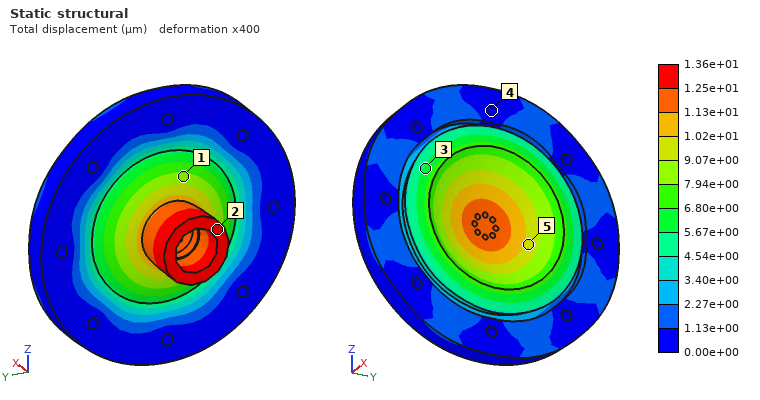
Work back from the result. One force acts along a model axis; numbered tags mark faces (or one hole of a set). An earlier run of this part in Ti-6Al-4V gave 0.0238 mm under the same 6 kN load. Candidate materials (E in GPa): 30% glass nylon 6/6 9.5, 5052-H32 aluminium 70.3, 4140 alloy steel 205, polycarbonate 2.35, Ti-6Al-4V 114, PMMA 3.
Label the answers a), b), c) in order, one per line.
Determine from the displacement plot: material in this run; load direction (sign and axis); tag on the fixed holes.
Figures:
a) 4140 alloy steel
b) +X
c) 4
